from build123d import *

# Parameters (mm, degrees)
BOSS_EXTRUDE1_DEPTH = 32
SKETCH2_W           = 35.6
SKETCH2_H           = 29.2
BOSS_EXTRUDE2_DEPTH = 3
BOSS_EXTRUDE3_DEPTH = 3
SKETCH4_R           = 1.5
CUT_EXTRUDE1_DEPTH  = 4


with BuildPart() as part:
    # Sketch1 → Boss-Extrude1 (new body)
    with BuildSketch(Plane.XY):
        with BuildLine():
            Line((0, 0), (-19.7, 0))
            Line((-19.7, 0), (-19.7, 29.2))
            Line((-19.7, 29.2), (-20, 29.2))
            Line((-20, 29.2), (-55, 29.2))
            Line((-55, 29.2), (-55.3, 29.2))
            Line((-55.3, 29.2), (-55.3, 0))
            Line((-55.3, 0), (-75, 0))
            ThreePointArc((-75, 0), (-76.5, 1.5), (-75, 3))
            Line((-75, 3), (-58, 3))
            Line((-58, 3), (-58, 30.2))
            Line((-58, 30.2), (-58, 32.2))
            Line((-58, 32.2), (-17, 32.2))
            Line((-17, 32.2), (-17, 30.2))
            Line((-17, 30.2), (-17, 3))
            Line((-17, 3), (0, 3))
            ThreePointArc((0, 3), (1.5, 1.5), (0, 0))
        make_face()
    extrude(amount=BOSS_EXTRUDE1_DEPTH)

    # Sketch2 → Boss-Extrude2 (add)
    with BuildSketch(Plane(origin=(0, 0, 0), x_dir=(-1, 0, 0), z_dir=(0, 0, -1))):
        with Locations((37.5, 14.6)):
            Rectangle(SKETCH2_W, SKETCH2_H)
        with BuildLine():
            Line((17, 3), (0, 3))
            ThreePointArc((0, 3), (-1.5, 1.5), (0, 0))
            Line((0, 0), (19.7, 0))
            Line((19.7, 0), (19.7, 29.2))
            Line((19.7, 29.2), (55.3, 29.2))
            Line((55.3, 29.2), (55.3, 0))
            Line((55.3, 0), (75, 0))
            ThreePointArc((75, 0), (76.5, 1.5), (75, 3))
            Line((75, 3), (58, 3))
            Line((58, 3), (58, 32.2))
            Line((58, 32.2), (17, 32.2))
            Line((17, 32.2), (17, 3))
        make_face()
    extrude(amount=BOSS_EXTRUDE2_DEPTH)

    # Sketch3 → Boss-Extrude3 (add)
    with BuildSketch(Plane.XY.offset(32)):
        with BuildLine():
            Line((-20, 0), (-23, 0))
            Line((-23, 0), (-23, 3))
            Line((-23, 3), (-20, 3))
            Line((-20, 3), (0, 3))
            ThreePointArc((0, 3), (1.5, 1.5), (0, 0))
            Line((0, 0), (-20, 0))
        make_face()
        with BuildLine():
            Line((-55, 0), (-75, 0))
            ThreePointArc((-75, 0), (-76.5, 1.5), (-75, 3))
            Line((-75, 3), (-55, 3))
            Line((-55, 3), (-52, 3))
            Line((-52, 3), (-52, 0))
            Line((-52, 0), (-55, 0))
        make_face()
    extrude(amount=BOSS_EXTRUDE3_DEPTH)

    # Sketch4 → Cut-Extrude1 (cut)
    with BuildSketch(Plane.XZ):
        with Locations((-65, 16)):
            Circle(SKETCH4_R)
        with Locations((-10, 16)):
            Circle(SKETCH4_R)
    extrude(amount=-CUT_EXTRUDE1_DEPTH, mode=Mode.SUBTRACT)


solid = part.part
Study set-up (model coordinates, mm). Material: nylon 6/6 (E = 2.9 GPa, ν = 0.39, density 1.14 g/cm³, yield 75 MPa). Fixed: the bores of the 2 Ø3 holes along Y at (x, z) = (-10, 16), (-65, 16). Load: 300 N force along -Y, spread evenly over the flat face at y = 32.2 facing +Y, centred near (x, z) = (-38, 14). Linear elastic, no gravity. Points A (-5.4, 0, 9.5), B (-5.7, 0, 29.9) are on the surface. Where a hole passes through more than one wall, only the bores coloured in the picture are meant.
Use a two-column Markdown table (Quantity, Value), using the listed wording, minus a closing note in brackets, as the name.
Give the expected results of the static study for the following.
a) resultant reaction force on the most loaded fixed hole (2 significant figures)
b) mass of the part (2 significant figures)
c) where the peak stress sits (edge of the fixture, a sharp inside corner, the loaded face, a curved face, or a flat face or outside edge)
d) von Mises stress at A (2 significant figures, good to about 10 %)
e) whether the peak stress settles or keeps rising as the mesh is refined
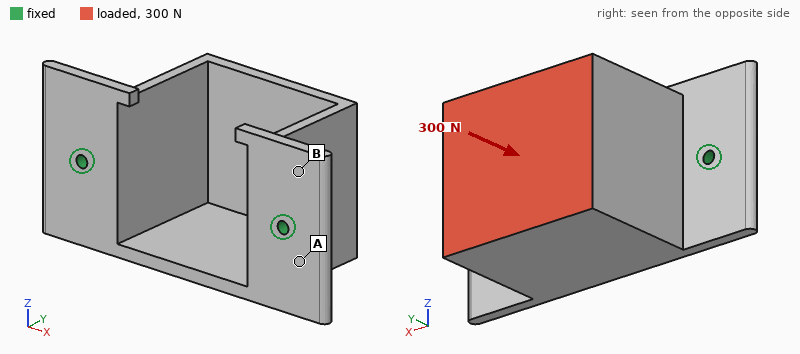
| Quantity | Value |
|---|---|
| resultant reaction force on the most loaded fixed hole | 150 N |
| mass of the part | 20 g |
| where the peak stress sits | edge of the fixture |
| von Mises stress at A | 4.4 MPa |
| whether the peak stress settles or keeps rising as the mesh is refined | keeps rising |
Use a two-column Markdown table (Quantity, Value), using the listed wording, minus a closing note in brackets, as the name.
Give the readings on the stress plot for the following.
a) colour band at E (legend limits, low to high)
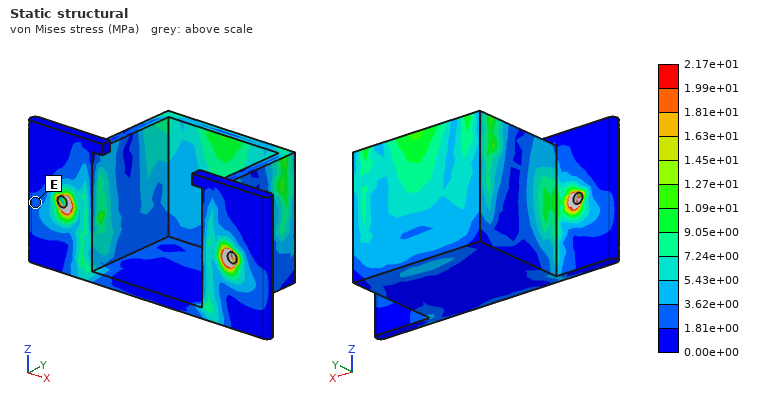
| Quantity | Value |
|---|---|
| colour band at E | 1.81e+00 to 3.62e+00 MPa |
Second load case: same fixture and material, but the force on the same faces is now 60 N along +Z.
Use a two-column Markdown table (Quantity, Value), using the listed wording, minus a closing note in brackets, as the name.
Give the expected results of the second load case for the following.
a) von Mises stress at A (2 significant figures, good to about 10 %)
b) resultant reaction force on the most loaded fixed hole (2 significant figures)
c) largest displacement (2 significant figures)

| Quantity | Value |
|---|---|
| von Mises stress at A | 7.8 MPa |
| resultant reaction force on the most loaded fixed hole | 33 N |
| largest displacement | 0.96 mm |
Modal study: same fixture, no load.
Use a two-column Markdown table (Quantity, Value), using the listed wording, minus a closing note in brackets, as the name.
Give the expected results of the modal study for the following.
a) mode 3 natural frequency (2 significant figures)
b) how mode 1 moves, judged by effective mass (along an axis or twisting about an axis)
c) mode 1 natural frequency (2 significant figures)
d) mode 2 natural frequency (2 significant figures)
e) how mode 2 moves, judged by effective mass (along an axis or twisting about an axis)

| Quantity | Value |
|---|---|
| mode 3 natural frequency | 1600 Hz |
| how mode 1 moves, judged by effective mass | along Z |
| mode 1 natural frequency | 440 Hz |
| mode 2 natural frequency | 710 Hz |
| how mode 2 moves, judged by effective mass | along X |
